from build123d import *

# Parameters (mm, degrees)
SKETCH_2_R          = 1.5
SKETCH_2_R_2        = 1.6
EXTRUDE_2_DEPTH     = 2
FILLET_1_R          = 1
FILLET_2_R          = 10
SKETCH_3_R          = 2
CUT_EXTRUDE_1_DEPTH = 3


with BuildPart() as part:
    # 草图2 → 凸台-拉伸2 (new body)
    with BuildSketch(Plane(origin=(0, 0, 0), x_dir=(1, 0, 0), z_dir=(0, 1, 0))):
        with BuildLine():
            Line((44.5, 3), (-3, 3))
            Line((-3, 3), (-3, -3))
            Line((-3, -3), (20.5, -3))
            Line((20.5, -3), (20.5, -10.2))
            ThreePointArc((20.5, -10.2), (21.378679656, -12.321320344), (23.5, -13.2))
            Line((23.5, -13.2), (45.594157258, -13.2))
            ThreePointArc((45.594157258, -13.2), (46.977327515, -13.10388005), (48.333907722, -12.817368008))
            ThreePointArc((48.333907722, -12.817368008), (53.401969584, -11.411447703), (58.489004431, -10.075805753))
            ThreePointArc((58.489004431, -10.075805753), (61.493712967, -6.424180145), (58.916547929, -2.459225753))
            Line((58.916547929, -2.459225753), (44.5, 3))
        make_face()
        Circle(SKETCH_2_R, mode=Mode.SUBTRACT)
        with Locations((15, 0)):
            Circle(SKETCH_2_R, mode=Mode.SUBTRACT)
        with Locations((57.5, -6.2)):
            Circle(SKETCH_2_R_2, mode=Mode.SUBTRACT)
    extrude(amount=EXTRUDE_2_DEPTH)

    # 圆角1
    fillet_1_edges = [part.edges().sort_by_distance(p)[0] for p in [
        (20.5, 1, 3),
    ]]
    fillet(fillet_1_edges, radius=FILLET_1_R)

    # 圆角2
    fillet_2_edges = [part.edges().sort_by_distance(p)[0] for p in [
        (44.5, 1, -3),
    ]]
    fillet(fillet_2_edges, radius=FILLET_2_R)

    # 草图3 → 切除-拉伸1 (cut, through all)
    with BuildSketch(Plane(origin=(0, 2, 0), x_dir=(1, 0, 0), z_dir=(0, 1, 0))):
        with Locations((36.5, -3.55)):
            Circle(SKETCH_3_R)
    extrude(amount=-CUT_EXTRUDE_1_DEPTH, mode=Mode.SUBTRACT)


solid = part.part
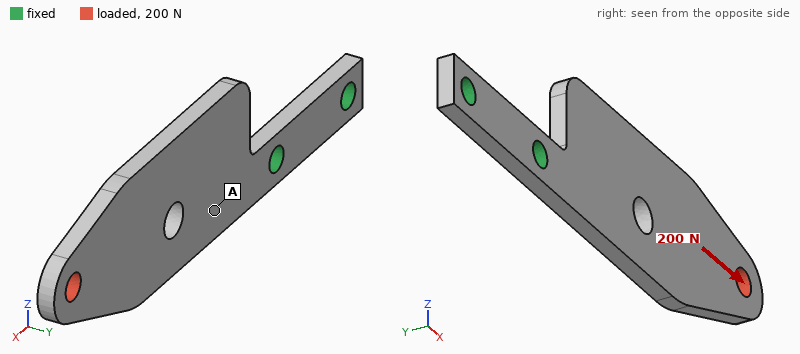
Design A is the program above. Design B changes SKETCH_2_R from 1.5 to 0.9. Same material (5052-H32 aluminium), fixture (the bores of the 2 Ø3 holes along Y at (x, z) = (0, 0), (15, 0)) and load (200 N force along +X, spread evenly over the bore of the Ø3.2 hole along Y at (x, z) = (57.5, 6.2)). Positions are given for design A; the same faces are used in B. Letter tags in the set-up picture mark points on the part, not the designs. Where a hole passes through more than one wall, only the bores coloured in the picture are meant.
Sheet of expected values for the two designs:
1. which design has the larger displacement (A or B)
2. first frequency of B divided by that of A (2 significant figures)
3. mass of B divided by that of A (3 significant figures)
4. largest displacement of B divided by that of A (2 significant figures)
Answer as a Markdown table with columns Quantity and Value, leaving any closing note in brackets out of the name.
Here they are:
| Quantity | Value |
|---|---|
| which design has the larger displacement | B |
| first frequency of B divided by that of A | 0.95 |
| mass of B divided by that of A | 1.01 |
| largest displacement of B divided by that of A | 1.2 |
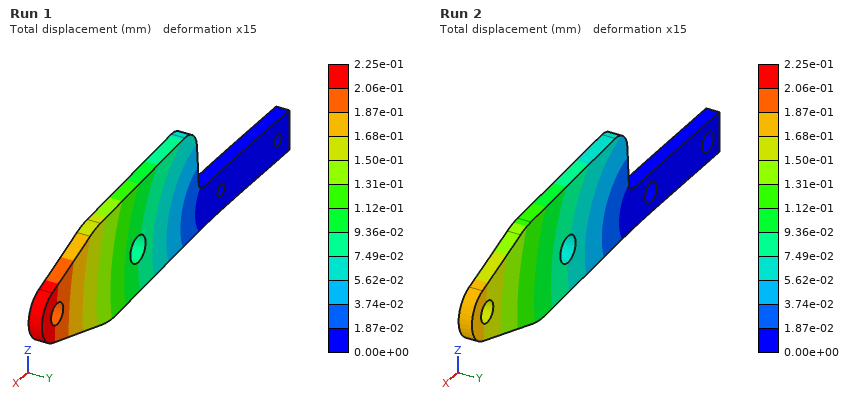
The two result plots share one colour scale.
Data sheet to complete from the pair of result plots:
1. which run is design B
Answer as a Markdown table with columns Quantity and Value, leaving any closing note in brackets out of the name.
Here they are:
| Quantity | Value |
|---|---|
| which run is design B | Run 1 |
